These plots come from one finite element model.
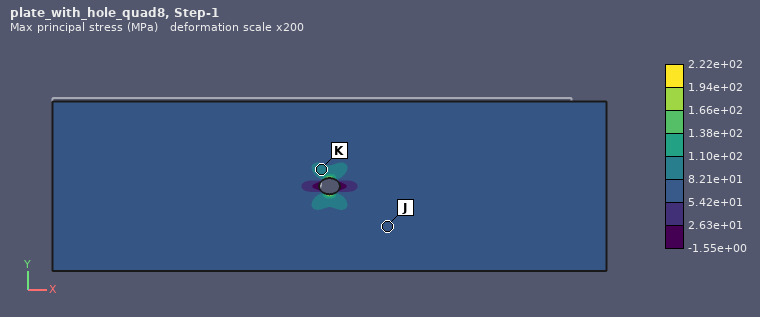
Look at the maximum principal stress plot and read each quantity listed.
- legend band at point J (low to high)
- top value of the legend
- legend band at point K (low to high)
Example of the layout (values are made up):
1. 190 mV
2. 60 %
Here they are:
1. 5.42e+01 to 8.21e+01 MPa
2. 2.22e+02 MPa
3. 8.21e+01 to 1.10e+02 MPa
